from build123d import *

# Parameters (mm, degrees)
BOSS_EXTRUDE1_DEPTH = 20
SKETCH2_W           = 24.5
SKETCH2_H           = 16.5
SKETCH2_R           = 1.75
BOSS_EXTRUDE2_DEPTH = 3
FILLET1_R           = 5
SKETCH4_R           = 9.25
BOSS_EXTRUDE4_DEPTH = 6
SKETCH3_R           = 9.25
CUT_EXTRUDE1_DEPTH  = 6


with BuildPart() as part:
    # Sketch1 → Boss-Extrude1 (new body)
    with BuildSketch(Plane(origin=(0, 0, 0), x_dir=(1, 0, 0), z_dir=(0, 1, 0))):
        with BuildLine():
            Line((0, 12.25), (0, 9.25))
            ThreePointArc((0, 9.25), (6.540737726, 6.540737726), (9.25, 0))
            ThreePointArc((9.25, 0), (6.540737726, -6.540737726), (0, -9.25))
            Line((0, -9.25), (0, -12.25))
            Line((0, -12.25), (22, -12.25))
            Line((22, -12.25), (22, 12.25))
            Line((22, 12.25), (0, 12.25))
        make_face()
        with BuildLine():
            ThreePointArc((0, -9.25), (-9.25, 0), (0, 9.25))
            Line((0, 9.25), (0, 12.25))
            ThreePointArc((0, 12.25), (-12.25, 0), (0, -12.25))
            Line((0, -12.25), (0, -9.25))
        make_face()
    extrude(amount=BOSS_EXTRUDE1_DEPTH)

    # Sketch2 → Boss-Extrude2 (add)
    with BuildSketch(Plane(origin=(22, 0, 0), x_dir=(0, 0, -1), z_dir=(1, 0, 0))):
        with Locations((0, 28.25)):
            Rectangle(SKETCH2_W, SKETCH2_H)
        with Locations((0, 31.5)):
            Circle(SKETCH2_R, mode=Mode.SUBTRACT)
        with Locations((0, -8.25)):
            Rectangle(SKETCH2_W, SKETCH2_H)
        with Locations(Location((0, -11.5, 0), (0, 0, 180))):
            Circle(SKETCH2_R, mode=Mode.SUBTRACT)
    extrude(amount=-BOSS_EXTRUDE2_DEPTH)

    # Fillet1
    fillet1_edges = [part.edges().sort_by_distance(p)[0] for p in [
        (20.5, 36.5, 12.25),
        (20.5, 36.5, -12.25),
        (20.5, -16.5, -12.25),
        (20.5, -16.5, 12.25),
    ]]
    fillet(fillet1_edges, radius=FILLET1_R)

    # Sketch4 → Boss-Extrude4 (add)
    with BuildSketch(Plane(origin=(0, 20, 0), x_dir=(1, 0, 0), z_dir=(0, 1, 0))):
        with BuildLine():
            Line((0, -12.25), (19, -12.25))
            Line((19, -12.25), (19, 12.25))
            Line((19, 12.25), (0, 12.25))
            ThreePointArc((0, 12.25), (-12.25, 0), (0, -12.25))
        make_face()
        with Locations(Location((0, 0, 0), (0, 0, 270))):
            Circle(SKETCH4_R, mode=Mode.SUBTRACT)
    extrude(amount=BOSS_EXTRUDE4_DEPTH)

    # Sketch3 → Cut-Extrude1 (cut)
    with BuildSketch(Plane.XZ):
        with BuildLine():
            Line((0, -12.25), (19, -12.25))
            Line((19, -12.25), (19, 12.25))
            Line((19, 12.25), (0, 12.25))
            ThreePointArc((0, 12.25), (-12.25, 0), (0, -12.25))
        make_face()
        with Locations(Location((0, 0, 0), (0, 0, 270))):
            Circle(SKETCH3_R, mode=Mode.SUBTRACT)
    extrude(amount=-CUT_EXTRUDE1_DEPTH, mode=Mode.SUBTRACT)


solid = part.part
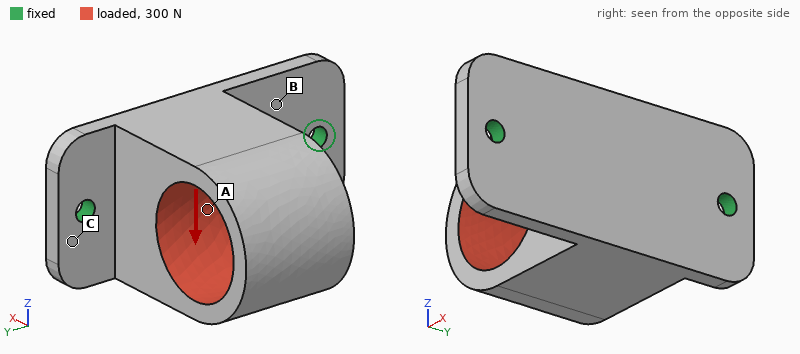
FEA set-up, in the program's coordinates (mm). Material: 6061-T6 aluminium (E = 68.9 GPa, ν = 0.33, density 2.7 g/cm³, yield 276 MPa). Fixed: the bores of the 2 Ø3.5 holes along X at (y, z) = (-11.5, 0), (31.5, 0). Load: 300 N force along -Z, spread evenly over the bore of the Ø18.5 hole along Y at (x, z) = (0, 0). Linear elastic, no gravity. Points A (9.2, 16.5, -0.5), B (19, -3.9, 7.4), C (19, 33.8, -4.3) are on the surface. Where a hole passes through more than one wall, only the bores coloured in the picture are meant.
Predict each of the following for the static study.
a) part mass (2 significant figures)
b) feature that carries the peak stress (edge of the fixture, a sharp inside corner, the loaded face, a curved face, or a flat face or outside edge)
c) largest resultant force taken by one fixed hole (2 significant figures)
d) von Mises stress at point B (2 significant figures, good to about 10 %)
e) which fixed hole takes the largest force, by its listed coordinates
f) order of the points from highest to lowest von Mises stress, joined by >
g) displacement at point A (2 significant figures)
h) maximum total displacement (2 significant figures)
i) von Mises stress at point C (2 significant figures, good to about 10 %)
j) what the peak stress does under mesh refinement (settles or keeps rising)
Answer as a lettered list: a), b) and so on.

a) 34 g
b) edge of the fixture
c) 200 N
d) 28 MPa
e) (31.5, 0)
f) C > B > A
g) 0.056 mm
h) 0.16 mm
i) 66 MPa
j) keeps rising
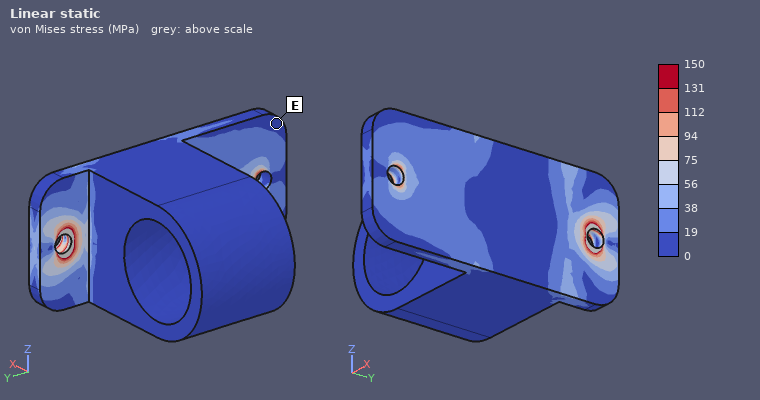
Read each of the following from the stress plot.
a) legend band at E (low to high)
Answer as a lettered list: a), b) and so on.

a) 0 to 19 MPa
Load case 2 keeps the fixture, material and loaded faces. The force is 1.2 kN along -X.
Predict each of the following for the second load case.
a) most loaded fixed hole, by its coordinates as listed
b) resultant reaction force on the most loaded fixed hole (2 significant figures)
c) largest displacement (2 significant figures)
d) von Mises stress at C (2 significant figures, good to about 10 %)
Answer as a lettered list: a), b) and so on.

a) (31.5, 0)
b) 810 N
c) 99 µm
d) 26 MPa
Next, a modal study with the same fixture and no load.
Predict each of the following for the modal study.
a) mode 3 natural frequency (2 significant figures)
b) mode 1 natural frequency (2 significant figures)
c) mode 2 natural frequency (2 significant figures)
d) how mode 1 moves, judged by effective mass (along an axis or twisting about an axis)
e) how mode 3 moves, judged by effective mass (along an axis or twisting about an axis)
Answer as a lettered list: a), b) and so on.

a) 8300 Hz
b) 2000 Hz
c) 3500 Hz
d) along Z
e) along X
